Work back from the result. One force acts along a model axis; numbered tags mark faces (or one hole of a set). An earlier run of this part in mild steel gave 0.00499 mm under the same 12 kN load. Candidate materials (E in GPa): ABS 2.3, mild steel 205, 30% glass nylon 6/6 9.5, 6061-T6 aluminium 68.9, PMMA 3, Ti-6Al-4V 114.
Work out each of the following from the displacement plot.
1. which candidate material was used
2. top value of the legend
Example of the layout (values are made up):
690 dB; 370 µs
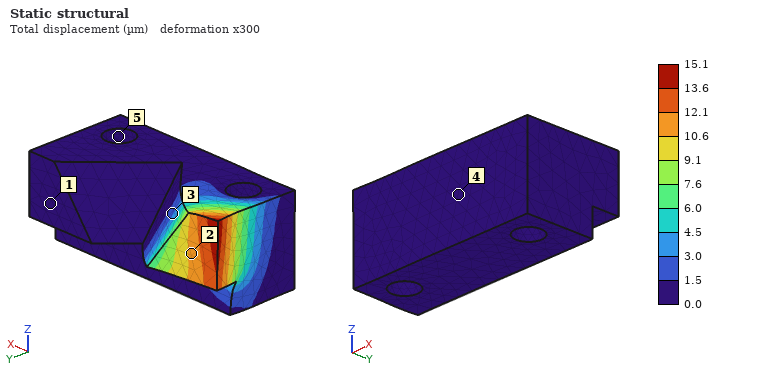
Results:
6061-T6 aluminium; 15.1 µm
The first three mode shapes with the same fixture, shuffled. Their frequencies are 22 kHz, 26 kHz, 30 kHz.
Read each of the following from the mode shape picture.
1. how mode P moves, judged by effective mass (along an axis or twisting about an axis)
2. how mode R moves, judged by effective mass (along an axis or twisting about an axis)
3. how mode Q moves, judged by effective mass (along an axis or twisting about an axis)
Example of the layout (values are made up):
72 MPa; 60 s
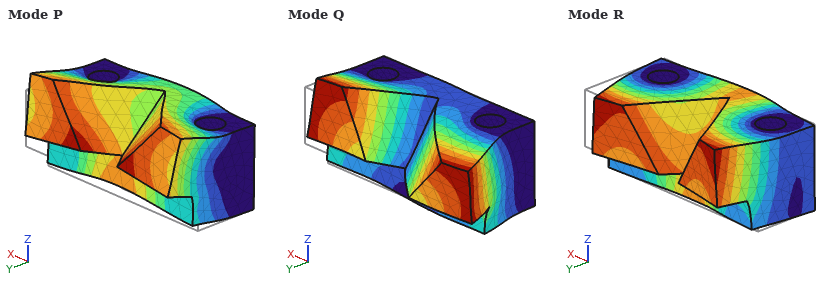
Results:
along Z; along Y; along X
